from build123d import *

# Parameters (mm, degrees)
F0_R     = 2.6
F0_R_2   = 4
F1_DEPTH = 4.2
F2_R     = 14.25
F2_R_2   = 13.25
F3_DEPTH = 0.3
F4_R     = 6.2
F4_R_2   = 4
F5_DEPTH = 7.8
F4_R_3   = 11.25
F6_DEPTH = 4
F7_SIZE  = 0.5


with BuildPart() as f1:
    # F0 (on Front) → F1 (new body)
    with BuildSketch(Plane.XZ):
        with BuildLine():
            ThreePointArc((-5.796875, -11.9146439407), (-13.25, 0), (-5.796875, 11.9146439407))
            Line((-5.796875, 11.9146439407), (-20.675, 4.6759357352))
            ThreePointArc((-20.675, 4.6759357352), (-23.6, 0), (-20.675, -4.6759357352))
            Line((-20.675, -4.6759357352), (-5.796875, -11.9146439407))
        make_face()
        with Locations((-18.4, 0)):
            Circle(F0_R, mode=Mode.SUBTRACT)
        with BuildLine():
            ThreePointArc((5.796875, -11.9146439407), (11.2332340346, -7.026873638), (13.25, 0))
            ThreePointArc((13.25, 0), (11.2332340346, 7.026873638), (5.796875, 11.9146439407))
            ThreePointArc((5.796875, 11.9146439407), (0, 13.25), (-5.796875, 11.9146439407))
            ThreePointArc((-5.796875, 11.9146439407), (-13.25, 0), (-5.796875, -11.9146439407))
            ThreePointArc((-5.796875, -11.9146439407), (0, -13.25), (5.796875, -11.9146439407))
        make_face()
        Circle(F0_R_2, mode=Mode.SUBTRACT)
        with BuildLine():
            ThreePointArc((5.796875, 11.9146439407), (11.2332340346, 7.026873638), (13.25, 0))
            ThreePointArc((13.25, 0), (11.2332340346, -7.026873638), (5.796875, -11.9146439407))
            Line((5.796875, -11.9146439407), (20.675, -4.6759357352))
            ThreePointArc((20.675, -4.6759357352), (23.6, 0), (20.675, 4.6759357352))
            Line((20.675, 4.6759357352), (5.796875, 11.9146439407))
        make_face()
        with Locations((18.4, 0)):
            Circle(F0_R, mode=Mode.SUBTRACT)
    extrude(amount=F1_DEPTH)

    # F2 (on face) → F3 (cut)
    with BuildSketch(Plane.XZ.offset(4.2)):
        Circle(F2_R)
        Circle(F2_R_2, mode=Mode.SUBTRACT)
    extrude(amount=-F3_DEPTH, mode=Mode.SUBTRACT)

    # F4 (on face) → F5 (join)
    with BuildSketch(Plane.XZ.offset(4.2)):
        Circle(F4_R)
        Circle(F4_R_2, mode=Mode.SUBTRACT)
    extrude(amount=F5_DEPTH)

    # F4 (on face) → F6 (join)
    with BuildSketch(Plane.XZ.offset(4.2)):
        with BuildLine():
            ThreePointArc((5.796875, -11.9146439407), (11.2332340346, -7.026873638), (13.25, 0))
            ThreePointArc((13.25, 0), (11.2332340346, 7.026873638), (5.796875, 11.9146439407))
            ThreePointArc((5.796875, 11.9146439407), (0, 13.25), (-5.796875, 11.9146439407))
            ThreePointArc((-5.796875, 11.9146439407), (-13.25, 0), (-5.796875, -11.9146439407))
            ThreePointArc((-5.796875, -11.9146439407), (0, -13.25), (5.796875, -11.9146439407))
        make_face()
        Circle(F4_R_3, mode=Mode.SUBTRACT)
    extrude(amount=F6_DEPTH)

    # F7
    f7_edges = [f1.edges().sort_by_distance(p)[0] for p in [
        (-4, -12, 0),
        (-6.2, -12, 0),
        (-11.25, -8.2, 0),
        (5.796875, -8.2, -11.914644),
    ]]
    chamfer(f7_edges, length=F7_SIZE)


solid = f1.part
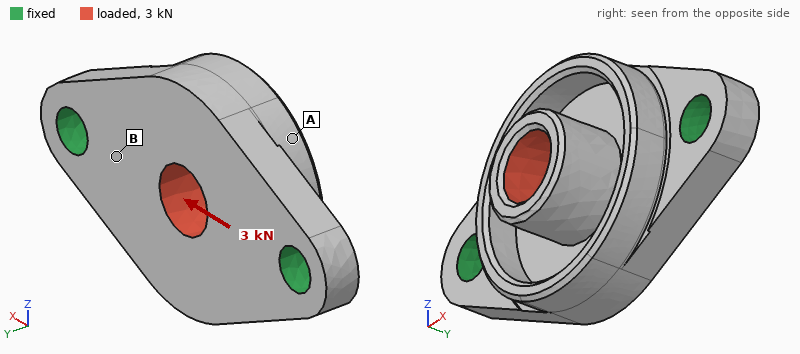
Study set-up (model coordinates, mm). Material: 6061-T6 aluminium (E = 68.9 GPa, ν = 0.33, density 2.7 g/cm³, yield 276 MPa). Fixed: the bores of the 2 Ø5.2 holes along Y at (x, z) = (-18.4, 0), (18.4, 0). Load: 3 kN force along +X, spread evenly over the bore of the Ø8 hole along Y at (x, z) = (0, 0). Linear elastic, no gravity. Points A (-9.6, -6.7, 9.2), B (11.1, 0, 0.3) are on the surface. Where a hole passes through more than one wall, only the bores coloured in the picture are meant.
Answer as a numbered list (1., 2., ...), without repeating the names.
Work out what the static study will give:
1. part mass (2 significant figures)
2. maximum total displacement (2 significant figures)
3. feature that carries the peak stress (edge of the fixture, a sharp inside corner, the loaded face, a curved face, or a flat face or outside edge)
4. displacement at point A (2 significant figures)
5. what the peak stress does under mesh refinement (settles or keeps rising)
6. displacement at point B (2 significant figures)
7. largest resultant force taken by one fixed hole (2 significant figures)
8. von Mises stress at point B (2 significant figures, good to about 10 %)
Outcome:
1. 11 g
2. 29 µm
3. edge of the fixture
4. 6.4 µm
5. keeps rising
6. 6.1 µm
7. 1.6 kN
8. 31 MPa
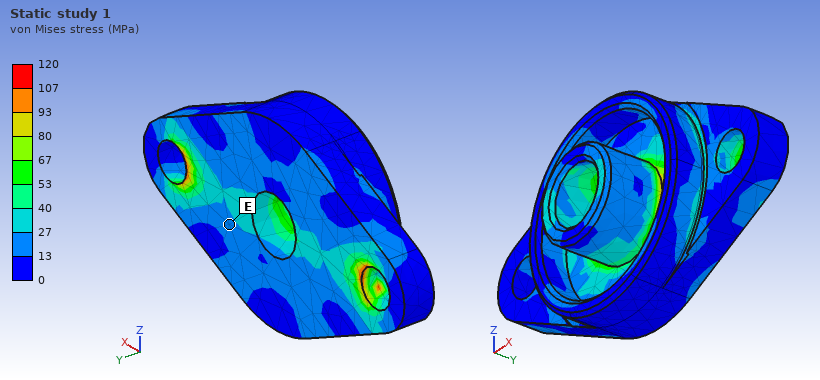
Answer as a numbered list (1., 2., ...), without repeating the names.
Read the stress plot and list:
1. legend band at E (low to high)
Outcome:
1. 13 to 27 MPa
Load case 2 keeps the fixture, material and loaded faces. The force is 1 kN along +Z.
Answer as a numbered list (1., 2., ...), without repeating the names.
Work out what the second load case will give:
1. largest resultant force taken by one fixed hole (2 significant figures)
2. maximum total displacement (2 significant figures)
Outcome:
1. 500 N
2. 28 µm
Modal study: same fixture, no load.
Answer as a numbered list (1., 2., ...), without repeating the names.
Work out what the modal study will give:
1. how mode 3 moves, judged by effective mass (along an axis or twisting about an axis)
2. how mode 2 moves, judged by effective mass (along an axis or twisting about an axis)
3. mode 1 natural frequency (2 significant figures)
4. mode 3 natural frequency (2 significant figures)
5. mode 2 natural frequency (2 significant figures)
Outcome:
1. along Z
2. along Y
3. 11 kHz
4. 28 kHz
5. 13 kHz
